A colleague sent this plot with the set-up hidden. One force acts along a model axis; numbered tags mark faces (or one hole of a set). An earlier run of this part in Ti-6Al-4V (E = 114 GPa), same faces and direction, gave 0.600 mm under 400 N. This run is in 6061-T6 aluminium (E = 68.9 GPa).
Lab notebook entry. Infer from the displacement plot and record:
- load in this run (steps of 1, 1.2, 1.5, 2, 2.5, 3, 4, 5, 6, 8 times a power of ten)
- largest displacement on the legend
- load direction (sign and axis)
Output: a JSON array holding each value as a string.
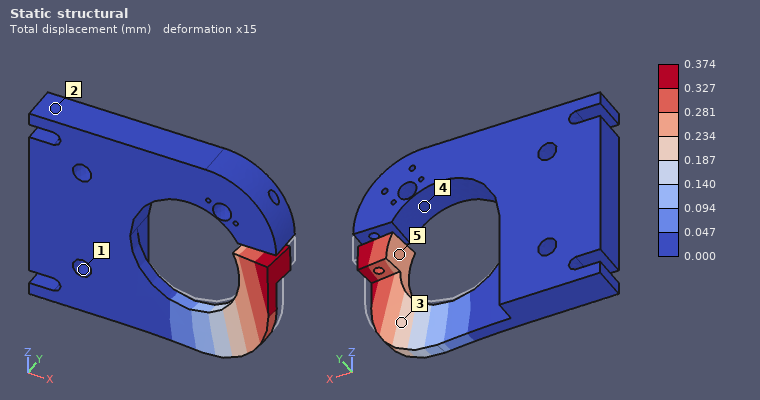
["150 N", "0.374 mm", "-Y"]
